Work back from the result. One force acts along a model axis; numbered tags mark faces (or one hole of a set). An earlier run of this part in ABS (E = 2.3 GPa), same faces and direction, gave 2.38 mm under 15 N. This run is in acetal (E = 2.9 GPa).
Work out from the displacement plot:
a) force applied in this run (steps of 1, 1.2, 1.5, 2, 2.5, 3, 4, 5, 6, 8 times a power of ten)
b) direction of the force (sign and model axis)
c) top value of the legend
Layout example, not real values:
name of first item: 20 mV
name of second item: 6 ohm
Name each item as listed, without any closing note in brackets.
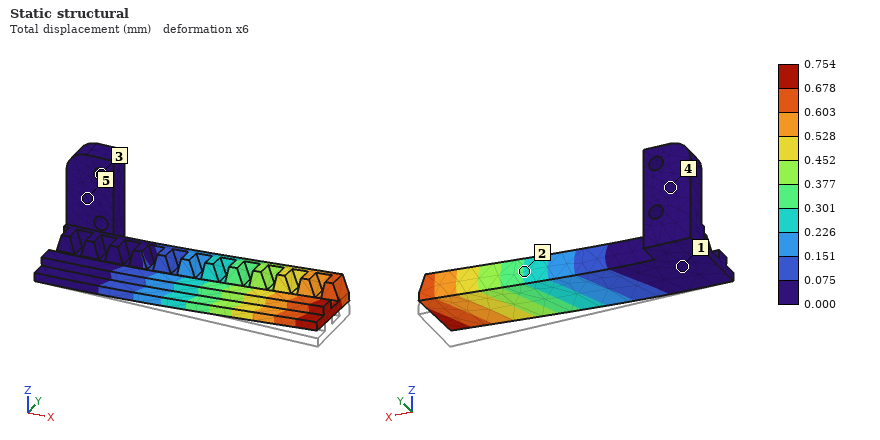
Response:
force applied in this run: 6 N
direction of the force: +Z
top value of the legend: 0.754 mm
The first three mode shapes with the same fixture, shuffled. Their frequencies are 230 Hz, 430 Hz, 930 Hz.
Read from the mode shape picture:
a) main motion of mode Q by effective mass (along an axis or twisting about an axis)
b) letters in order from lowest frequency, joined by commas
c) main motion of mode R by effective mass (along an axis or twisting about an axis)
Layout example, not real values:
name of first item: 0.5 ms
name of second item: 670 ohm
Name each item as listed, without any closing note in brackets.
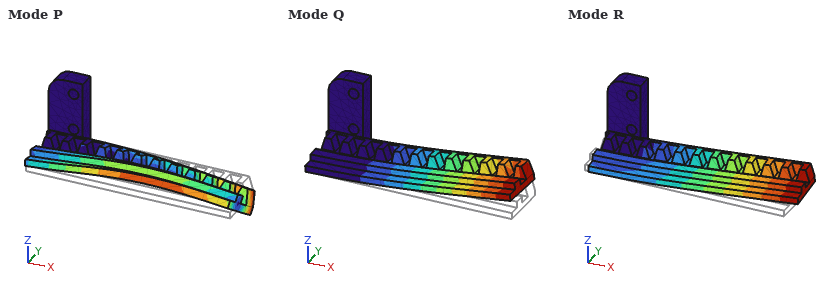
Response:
main motion of mode Q by effective mass: along Z
letters in order from lowest frequency, joined by commas: Q, R, P
main motion of mode R by effective mass: along Y
